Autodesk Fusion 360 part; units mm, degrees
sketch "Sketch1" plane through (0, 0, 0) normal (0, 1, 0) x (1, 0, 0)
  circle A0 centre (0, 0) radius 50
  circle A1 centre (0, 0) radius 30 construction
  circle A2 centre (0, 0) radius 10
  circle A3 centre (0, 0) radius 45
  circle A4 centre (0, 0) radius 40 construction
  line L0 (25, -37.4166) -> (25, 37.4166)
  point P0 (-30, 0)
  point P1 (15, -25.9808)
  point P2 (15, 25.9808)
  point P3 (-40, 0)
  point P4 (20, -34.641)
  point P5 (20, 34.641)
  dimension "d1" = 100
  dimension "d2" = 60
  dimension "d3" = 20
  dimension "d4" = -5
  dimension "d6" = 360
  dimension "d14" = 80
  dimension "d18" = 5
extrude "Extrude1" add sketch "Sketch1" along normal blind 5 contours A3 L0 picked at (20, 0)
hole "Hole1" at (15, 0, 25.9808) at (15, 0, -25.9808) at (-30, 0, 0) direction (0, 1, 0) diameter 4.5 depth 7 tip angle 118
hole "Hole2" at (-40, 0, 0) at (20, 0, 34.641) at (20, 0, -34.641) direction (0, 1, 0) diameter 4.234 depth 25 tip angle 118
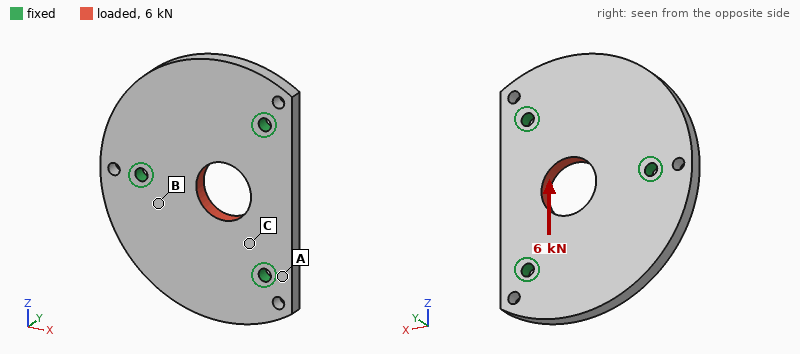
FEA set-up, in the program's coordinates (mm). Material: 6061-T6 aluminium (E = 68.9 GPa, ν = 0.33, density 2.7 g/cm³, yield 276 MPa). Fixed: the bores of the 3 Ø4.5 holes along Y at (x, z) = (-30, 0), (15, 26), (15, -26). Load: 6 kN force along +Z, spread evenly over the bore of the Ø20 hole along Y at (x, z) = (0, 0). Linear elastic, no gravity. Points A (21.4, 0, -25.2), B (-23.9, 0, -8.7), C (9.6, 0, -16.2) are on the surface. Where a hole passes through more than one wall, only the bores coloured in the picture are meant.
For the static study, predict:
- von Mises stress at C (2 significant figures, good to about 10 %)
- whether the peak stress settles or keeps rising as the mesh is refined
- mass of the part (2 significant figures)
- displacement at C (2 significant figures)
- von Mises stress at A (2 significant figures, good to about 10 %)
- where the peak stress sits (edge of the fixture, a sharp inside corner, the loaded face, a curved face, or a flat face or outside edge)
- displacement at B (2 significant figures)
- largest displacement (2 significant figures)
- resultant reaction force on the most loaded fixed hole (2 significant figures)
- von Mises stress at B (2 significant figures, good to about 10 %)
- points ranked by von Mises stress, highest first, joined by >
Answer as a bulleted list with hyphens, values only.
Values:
- 22 MPa
- keeps rising
- 66 g
- 4.3 µm
- 5.6 MPa
- edge of the fixture
- 4.0 µm
- 11 µm
- 2.0 kN
- 14 MPa
- C > B > A
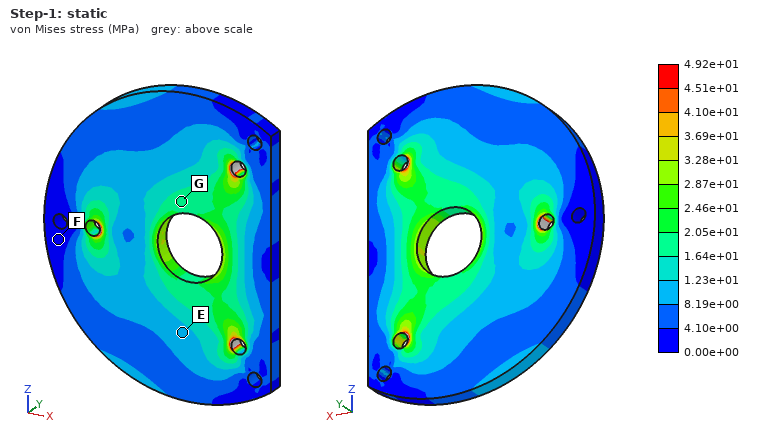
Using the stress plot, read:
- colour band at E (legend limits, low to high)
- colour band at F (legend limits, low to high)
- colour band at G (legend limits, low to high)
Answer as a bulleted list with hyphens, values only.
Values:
- 8.19e+00 to 1.23e+01 MPa
- 0.00e+00 to 4.10e+00 MPa
- 1.64e+01 to 2.05e+01 MPa
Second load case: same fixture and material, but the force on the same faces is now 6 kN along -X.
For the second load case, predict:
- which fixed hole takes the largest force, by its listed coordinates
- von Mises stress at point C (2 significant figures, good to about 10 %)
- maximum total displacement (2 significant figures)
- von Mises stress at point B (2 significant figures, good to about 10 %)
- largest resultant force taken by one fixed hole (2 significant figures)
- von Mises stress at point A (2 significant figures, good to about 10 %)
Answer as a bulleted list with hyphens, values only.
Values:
- (-30, 0)
- 18 MPa
- 17 µm
- 13 MPa
- 2.2 kN
- 12 MPa
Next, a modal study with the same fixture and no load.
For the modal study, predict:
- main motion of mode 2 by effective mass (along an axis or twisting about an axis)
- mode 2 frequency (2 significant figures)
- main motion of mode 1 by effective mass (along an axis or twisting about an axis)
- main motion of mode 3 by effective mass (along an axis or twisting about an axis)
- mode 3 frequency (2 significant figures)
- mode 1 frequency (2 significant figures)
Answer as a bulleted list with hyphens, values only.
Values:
- along Y
- 4500 Hz
- twisting about X
- along Y
- 9000 Hz
- 4100 Hz
